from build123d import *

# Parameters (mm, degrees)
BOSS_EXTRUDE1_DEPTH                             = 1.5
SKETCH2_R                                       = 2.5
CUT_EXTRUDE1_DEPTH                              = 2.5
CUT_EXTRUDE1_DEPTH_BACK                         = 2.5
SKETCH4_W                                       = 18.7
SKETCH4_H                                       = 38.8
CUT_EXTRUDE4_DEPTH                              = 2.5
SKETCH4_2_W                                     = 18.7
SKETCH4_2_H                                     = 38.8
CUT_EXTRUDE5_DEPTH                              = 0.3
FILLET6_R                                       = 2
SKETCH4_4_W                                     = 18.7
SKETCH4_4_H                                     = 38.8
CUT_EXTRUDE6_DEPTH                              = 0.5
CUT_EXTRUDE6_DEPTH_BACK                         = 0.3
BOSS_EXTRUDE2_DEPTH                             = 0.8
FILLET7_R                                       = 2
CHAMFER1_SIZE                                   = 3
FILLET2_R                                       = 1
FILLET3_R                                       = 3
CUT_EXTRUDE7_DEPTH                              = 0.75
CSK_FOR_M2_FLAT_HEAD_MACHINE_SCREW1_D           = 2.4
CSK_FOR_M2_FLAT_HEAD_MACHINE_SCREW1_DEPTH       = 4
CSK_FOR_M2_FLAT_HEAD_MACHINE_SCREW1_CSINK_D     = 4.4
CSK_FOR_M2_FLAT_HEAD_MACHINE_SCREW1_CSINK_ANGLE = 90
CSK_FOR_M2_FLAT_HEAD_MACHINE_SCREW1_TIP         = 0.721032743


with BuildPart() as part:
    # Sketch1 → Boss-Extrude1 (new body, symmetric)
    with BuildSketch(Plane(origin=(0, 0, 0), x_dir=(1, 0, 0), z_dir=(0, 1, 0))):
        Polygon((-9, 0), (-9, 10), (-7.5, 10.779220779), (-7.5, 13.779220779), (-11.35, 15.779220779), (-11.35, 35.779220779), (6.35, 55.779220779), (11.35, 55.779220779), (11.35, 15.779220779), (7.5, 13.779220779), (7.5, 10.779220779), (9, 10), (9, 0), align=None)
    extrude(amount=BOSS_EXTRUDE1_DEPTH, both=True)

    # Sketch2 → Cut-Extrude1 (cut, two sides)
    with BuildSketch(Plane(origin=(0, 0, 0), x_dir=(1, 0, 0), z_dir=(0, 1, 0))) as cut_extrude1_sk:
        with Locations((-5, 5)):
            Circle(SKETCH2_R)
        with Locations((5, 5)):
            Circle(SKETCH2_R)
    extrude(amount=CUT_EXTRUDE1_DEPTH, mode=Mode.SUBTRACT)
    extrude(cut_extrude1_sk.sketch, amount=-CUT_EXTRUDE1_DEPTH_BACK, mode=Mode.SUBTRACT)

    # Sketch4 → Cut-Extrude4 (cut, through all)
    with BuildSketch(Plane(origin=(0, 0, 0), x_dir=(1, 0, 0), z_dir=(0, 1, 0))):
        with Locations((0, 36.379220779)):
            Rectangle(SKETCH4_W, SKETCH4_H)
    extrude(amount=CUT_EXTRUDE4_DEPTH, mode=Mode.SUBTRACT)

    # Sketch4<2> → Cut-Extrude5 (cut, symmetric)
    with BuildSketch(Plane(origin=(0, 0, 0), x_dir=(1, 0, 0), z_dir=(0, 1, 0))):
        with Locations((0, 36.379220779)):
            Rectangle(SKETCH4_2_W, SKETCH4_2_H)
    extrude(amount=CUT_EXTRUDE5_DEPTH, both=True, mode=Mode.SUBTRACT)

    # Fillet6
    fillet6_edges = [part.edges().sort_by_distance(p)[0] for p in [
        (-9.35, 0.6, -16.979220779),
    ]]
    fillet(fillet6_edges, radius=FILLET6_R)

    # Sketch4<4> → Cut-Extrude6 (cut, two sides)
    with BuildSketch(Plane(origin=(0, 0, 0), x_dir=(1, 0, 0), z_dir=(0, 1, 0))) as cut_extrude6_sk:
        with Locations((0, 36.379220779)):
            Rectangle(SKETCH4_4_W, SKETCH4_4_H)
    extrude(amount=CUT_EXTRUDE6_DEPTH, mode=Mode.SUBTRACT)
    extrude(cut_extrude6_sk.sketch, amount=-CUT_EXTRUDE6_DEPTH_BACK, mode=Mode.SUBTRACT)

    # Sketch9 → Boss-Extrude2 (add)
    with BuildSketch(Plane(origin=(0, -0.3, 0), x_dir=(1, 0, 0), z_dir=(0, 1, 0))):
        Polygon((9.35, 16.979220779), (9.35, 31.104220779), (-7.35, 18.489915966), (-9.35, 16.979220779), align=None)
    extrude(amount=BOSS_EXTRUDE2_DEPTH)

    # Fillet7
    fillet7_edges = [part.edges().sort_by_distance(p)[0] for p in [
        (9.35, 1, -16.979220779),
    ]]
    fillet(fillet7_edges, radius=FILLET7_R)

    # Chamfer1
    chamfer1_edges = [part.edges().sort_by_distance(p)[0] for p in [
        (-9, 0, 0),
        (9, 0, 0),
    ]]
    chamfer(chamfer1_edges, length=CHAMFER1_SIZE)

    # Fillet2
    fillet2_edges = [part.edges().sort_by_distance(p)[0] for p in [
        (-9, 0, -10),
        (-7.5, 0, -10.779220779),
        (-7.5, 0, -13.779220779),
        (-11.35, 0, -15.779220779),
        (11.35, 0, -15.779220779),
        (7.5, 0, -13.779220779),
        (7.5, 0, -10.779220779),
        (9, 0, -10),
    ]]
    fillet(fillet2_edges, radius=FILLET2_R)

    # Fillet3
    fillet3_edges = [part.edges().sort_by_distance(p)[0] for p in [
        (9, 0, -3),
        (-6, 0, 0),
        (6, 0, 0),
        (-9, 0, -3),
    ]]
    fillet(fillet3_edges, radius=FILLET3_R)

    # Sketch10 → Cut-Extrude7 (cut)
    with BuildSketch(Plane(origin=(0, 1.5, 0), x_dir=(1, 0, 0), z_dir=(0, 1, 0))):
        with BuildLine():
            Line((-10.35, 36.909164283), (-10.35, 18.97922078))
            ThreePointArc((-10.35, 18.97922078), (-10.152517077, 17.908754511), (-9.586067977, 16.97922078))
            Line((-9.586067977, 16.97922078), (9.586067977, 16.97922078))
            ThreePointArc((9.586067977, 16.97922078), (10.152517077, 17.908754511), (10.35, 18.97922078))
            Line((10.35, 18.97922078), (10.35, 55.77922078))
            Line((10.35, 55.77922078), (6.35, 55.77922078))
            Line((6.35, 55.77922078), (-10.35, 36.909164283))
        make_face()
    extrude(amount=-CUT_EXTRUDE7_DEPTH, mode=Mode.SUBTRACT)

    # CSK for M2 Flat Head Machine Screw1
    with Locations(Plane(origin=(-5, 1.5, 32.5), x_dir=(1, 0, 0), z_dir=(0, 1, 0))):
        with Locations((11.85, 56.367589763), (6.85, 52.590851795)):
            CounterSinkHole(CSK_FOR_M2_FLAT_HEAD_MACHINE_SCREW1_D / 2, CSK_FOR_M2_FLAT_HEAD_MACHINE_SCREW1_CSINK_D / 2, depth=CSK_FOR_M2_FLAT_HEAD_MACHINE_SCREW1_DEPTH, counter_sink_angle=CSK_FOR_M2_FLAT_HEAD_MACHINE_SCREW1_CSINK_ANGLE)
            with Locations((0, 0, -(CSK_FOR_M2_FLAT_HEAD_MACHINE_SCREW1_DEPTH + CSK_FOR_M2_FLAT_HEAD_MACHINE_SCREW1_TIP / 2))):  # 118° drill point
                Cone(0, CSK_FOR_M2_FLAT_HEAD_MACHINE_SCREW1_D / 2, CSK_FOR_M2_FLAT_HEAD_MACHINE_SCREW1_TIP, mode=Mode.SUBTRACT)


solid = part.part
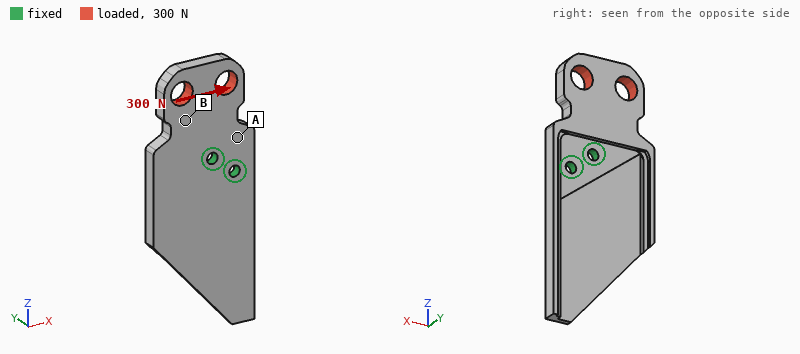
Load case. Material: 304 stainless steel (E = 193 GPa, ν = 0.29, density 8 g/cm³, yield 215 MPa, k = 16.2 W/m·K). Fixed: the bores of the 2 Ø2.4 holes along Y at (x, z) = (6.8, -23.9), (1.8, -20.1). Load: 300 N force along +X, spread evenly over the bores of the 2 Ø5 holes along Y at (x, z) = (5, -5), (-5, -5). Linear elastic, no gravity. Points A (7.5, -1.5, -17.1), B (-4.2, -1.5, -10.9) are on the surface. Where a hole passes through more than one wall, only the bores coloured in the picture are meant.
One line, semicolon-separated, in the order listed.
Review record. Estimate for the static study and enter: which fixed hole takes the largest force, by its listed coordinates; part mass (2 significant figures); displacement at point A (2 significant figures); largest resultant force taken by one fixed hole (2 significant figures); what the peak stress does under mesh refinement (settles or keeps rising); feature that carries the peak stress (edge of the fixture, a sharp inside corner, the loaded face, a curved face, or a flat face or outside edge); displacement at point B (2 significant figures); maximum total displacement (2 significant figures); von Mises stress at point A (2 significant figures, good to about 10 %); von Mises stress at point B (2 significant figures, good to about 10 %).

(1.8, -20.1); 15 g; 2.0 µm; 690 N; keeps rising; edge of the fixture; 5.7 µm; 12 µm; 36 MPa; 17 MPa
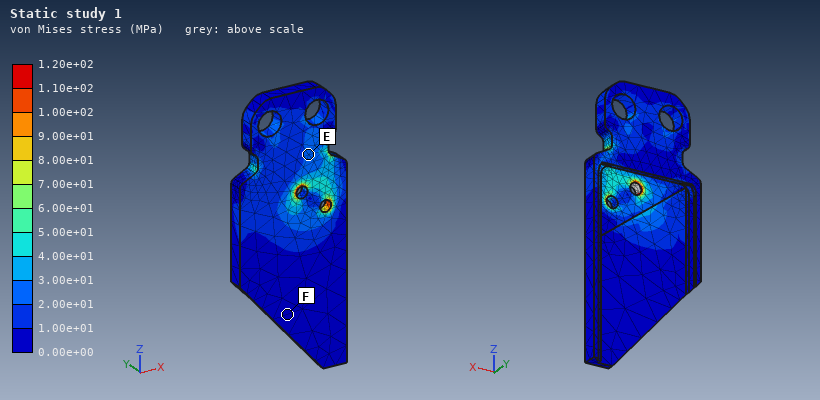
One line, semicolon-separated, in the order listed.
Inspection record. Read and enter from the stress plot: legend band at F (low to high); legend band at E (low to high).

0.00e+00 to 1.00e+01 MPa; 2.00e+01 to 3.00e+01 MPa
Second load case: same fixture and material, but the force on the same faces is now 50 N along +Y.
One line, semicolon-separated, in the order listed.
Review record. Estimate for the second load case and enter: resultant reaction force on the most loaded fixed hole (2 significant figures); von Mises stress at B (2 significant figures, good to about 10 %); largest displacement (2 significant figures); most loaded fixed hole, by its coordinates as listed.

83 N; 10 MPa; 28 µm; (1.8, -20.1)
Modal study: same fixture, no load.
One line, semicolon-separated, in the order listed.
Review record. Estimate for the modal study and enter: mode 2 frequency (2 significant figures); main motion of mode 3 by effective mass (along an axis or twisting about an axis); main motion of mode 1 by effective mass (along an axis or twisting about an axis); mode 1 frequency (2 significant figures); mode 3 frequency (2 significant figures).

3900 Hz; along Y; along Y; 2100 Hz; 4800 Hz
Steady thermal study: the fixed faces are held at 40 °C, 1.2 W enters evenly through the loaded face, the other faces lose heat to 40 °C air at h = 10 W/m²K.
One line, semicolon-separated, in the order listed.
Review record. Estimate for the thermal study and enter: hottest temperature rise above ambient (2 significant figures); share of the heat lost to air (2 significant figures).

30 K; 15 %
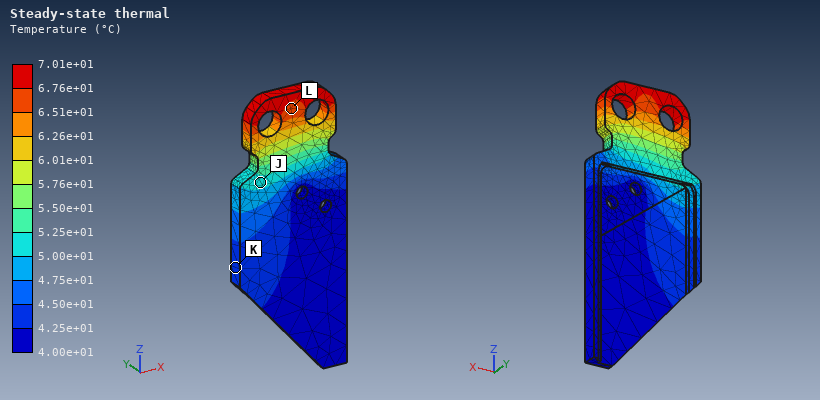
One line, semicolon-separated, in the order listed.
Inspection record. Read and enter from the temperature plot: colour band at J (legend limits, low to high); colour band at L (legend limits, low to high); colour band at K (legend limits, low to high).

5.00e+01 to 5.25e+01 °C; 6.51e+01 to 6.76e+01 °C; 4.25e+01 to 4.50e+01 °C
